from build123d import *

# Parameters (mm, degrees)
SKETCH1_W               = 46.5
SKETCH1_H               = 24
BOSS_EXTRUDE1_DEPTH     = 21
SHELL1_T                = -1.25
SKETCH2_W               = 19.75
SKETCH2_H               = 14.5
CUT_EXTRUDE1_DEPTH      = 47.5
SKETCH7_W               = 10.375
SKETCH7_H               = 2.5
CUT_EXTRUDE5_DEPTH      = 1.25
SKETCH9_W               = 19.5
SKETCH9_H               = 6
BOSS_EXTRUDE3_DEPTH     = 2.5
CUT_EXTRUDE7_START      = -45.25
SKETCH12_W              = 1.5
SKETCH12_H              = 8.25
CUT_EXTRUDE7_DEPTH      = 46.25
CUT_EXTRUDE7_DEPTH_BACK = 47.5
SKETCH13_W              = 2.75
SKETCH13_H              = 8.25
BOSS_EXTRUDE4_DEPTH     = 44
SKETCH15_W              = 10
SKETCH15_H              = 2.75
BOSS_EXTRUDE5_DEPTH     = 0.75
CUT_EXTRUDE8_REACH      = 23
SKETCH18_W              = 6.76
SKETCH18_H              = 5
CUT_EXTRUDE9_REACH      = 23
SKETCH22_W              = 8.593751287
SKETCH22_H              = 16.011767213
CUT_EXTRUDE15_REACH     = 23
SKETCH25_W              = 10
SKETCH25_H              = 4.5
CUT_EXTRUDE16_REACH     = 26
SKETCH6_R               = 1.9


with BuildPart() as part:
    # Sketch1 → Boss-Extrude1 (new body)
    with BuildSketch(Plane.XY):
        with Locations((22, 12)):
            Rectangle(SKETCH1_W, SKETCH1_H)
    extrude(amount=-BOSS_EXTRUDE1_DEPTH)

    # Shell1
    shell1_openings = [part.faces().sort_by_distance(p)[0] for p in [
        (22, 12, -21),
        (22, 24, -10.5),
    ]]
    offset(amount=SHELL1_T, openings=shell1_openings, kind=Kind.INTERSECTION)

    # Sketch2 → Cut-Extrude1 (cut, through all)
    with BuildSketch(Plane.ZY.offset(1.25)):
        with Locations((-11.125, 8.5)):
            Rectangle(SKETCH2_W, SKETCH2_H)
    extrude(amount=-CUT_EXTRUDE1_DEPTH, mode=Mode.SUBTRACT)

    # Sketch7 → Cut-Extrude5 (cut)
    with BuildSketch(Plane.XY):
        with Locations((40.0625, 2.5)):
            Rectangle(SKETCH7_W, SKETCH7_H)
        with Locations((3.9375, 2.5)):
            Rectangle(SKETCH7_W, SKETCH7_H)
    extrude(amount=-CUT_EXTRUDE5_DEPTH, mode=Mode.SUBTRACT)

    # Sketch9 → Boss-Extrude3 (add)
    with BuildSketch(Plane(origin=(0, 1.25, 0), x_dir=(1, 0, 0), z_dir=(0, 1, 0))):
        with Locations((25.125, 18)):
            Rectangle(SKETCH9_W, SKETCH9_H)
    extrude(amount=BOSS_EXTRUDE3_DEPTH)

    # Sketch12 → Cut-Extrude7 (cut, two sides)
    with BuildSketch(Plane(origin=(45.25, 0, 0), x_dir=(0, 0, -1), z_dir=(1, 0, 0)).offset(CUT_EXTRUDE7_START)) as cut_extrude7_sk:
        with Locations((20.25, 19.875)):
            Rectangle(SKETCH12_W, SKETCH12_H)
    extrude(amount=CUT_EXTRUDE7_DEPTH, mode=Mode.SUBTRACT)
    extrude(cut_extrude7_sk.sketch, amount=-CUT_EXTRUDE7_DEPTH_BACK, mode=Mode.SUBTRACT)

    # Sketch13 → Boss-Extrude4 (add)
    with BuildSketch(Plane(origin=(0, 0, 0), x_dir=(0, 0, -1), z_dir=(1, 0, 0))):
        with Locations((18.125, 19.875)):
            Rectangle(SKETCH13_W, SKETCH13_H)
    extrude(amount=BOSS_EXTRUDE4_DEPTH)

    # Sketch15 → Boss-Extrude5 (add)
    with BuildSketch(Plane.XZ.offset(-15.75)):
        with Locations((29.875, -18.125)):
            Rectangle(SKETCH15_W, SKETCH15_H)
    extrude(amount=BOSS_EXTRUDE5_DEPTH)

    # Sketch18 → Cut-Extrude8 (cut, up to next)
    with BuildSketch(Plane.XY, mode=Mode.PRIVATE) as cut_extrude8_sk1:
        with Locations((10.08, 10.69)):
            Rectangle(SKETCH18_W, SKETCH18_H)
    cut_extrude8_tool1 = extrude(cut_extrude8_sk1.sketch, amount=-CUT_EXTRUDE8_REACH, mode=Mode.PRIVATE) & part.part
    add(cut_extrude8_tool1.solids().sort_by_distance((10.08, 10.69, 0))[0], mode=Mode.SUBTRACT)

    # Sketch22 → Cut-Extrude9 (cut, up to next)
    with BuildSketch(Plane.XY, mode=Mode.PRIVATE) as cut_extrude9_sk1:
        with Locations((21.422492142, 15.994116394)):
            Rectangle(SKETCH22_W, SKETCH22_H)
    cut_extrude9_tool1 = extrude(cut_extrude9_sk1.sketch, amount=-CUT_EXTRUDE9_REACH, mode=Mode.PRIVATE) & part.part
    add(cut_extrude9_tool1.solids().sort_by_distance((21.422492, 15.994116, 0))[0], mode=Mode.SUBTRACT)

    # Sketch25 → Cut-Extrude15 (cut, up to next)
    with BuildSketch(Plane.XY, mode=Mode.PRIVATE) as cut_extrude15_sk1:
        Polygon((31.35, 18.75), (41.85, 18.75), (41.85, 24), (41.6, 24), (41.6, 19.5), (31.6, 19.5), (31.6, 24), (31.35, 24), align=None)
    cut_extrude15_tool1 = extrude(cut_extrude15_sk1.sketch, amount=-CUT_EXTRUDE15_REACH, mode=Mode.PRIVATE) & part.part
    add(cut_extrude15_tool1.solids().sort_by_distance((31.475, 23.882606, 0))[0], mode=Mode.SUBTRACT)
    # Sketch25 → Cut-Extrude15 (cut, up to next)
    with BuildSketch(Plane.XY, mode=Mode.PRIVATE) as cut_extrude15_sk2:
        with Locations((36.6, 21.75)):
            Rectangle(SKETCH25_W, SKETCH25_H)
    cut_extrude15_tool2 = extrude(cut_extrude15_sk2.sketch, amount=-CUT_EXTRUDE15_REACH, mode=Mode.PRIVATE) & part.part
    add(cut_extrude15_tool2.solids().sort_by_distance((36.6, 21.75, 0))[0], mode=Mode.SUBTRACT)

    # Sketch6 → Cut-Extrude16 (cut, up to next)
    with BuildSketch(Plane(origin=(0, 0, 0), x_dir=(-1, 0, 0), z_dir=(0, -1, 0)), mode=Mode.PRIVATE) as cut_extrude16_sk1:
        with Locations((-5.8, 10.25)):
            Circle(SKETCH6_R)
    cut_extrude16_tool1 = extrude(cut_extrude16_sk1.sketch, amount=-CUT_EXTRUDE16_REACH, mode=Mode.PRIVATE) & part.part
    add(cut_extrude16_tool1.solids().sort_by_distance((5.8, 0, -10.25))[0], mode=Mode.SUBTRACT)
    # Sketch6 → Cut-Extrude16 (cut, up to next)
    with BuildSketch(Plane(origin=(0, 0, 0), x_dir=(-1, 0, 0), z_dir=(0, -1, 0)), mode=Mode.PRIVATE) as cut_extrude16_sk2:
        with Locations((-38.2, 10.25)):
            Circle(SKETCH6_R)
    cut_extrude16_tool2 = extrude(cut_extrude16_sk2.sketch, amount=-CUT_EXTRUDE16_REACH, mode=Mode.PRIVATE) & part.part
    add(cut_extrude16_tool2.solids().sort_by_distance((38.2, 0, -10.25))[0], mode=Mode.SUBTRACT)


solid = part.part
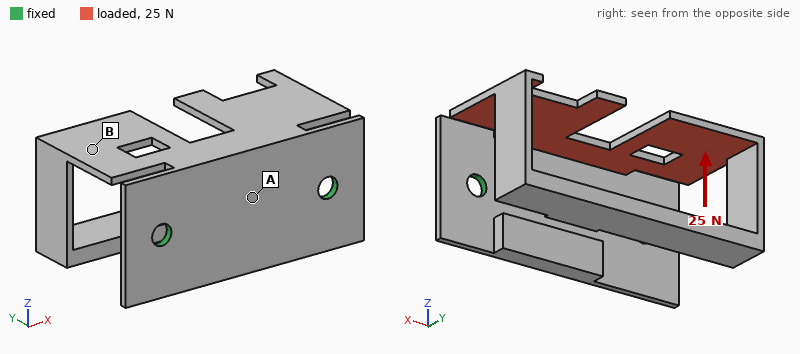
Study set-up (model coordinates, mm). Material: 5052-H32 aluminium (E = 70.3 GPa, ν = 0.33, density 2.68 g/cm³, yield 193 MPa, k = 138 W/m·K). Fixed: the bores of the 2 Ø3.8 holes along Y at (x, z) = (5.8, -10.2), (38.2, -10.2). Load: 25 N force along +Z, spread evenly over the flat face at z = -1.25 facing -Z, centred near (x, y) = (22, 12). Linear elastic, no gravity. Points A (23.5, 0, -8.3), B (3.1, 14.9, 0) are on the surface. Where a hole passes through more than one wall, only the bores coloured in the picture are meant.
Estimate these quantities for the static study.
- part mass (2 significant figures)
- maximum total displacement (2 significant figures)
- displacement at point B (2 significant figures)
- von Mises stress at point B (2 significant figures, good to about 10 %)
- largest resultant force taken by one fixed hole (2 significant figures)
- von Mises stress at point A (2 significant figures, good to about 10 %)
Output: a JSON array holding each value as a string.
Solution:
["10 g", "0.37 mm", "0.18 mm", "5.3 MPa", "13 N", "15 MPa"]
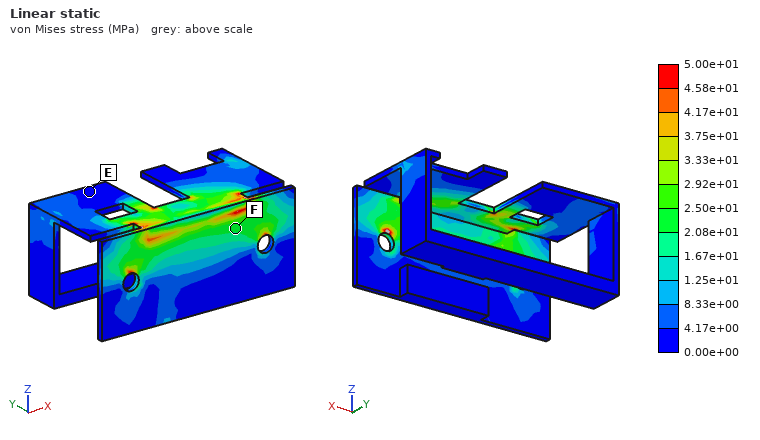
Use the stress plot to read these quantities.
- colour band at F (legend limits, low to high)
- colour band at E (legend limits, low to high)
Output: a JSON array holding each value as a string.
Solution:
["2.08e+01 to 2.50e+01 MPa", "0.00e+00 to 4.17e+00 MPa"]
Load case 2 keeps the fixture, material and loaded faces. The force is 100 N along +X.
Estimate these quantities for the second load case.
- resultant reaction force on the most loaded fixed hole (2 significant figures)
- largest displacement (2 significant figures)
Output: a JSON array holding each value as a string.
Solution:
["70 N", "0.18 mm"]
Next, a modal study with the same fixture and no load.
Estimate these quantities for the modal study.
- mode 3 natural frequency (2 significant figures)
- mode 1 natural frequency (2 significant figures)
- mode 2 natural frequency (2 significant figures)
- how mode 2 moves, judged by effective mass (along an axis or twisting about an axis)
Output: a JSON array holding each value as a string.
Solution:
["1100 Hz", "400 Hz", "650 Hz", "along X"]
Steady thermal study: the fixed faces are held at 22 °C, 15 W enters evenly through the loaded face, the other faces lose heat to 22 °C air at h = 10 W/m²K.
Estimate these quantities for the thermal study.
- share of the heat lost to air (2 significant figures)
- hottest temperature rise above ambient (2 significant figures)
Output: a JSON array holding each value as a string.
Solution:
["12 %", "73 K"]
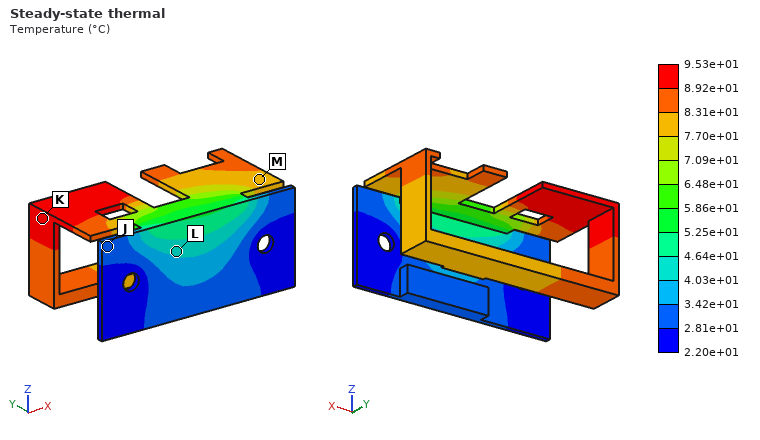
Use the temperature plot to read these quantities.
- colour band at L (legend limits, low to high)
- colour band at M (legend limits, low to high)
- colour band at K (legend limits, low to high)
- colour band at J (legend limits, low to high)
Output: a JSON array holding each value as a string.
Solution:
["4.03e+01 to 4.64e+01 °C", "7.70e+01 to 8.31e+01 °C", "8.92e+01 to 9.53e+01 °C", "2.81e+01 to 3.42e+01 °C"]
